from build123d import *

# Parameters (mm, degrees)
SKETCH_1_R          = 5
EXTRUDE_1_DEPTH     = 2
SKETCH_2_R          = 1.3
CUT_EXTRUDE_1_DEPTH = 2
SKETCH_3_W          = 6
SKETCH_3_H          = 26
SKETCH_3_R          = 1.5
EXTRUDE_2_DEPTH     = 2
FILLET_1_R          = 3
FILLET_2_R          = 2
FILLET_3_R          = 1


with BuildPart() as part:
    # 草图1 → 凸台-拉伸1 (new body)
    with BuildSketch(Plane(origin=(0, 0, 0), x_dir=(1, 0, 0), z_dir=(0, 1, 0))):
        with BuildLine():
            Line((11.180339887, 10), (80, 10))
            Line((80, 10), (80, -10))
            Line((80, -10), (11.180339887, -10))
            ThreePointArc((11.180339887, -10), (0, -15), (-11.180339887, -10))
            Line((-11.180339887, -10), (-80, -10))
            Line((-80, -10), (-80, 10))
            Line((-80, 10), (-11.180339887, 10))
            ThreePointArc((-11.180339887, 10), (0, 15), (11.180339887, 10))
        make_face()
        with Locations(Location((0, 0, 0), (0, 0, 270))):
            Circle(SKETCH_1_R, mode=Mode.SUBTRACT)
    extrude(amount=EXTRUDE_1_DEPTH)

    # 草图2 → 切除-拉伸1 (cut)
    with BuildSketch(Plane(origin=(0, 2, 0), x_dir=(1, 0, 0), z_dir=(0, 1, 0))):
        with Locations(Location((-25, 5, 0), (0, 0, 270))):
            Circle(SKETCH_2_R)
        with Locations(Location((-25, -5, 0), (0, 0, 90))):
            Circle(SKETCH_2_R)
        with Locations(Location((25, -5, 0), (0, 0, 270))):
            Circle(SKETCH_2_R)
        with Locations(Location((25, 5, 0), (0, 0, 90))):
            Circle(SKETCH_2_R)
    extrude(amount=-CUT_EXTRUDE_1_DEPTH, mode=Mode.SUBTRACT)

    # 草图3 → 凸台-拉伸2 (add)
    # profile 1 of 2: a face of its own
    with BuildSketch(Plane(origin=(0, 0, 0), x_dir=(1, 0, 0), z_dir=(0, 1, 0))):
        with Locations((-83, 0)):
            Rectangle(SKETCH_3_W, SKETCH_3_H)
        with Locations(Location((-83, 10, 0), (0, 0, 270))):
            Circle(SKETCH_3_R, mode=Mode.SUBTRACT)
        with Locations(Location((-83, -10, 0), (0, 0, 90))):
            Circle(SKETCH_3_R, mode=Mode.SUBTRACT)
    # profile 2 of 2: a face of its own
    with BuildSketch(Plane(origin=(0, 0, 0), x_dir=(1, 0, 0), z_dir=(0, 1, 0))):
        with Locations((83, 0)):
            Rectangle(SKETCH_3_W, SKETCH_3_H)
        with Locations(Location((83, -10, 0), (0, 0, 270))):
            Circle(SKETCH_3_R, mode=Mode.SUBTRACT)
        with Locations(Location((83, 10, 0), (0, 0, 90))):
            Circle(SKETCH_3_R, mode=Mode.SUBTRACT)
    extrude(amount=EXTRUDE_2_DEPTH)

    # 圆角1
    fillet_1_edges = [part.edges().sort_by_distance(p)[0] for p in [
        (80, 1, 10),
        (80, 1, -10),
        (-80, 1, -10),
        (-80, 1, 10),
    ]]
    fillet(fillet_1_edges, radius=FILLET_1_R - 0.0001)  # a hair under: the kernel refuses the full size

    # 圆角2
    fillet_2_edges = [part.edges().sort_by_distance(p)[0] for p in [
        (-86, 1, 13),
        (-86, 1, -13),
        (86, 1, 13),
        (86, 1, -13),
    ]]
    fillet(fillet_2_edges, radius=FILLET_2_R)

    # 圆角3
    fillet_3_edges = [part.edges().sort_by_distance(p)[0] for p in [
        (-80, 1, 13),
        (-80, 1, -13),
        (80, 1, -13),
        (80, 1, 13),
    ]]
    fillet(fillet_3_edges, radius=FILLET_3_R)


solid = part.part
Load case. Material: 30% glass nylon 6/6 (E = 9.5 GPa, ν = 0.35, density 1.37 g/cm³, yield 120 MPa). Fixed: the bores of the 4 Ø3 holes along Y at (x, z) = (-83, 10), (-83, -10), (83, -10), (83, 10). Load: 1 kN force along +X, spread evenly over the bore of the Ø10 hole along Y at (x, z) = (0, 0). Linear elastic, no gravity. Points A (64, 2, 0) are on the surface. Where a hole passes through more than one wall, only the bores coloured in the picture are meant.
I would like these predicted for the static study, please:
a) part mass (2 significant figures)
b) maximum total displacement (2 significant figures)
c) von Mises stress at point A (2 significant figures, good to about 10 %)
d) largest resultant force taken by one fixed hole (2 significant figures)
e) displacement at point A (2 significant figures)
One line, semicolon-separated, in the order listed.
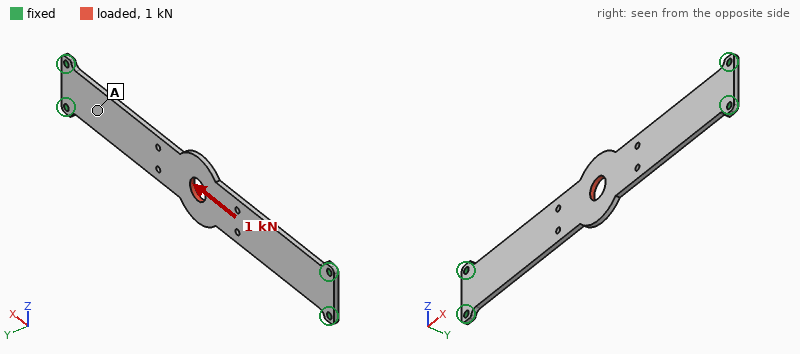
9.7 g; 0.12 mm; 12 MPa; 270 N; 0.033 mm
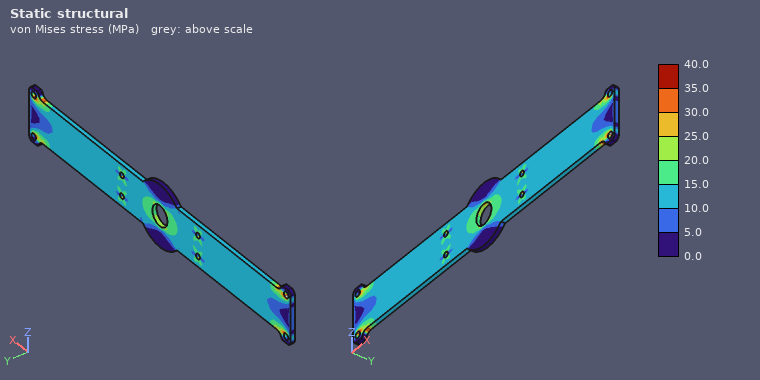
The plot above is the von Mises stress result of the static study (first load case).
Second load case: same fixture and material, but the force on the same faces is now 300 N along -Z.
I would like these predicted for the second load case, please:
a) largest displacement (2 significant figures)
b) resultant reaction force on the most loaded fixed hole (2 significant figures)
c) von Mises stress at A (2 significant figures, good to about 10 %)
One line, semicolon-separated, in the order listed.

0.56 mm; 320 N; 9.8 MPa
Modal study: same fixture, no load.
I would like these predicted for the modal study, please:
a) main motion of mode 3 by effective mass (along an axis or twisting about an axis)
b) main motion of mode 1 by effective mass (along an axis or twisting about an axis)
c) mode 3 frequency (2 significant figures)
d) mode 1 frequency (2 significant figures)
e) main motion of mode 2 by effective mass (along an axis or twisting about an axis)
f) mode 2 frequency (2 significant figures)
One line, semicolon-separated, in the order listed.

twisting about X; along Y; 850 Hz; 190 Hz; twisting about Z; 540 Hz
